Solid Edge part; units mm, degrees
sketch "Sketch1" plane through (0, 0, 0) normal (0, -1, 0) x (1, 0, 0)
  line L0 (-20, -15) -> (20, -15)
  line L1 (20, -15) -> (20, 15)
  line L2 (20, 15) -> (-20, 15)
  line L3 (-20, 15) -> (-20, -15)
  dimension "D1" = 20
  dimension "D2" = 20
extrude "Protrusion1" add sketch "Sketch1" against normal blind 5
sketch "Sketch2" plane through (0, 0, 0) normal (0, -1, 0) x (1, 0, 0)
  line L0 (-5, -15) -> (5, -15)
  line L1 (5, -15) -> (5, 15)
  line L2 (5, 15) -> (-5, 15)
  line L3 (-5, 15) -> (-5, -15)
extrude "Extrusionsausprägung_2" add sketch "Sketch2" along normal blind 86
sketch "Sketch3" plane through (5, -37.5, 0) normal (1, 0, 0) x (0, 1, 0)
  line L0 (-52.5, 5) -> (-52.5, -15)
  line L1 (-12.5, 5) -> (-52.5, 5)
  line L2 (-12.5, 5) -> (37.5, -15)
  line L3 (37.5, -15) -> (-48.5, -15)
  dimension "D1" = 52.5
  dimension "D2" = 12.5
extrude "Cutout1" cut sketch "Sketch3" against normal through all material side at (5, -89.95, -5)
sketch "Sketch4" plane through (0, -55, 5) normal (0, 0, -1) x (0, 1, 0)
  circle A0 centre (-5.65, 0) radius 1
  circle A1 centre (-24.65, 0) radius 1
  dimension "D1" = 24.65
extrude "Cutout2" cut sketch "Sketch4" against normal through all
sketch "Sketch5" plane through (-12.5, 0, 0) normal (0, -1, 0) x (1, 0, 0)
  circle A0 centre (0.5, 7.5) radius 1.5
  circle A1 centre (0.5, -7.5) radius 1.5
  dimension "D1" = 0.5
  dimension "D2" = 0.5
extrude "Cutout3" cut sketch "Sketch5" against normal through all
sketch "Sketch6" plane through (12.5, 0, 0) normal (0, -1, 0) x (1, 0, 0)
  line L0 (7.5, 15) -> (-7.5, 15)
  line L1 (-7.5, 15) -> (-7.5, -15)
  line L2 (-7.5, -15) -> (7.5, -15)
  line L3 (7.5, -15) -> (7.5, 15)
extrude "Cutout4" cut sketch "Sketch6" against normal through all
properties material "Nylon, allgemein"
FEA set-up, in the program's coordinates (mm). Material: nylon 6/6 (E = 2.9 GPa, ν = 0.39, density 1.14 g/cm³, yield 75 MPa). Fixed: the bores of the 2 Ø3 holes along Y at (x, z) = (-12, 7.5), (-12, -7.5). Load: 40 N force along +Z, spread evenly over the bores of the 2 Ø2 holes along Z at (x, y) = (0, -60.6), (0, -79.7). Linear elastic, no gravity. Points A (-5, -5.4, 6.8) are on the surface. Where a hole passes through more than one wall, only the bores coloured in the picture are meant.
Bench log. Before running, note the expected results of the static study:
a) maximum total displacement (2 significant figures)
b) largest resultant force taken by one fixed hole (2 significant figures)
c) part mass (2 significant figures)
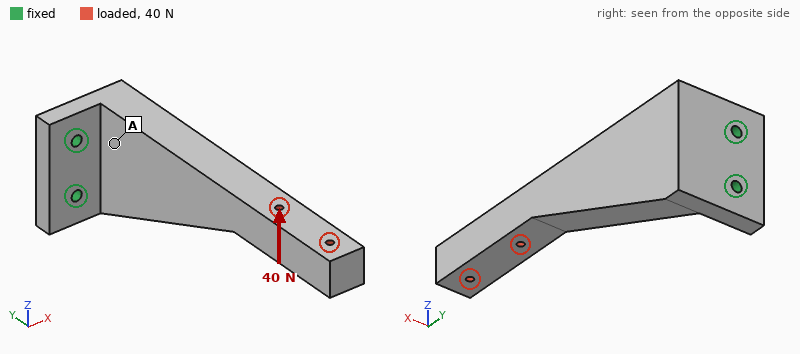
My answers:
1.1 mm
150 N
20 g
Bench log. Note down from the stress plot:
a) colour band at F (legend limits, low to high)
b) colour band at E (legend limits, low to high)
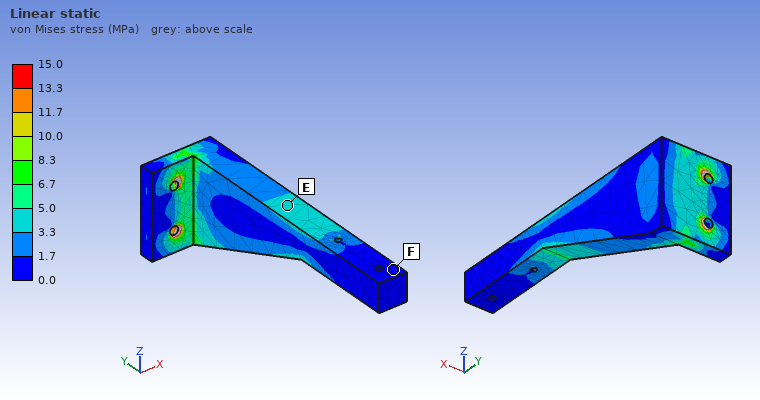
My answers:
0.0 to 1.7 MPa
3.3 to 5.0 MPa
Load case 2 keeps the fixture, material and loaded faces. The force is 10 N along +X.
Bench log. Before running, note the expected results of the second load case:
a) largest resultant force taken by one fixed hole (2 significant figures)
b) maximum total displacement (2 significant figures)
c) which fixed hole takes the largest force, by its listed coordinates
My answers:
12 N
1.0 mm
(-12, 7.5)
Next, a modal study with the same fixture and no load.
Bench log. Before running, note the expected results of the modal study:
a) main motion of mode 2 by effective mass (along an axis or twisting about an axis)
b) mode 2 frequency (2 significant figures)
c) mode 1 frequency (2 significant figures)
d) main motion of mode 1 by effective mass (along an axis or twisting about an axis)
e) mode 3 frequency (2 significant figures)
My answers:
along Z
510 Hz
250 Hz
along X
1400 Hz
